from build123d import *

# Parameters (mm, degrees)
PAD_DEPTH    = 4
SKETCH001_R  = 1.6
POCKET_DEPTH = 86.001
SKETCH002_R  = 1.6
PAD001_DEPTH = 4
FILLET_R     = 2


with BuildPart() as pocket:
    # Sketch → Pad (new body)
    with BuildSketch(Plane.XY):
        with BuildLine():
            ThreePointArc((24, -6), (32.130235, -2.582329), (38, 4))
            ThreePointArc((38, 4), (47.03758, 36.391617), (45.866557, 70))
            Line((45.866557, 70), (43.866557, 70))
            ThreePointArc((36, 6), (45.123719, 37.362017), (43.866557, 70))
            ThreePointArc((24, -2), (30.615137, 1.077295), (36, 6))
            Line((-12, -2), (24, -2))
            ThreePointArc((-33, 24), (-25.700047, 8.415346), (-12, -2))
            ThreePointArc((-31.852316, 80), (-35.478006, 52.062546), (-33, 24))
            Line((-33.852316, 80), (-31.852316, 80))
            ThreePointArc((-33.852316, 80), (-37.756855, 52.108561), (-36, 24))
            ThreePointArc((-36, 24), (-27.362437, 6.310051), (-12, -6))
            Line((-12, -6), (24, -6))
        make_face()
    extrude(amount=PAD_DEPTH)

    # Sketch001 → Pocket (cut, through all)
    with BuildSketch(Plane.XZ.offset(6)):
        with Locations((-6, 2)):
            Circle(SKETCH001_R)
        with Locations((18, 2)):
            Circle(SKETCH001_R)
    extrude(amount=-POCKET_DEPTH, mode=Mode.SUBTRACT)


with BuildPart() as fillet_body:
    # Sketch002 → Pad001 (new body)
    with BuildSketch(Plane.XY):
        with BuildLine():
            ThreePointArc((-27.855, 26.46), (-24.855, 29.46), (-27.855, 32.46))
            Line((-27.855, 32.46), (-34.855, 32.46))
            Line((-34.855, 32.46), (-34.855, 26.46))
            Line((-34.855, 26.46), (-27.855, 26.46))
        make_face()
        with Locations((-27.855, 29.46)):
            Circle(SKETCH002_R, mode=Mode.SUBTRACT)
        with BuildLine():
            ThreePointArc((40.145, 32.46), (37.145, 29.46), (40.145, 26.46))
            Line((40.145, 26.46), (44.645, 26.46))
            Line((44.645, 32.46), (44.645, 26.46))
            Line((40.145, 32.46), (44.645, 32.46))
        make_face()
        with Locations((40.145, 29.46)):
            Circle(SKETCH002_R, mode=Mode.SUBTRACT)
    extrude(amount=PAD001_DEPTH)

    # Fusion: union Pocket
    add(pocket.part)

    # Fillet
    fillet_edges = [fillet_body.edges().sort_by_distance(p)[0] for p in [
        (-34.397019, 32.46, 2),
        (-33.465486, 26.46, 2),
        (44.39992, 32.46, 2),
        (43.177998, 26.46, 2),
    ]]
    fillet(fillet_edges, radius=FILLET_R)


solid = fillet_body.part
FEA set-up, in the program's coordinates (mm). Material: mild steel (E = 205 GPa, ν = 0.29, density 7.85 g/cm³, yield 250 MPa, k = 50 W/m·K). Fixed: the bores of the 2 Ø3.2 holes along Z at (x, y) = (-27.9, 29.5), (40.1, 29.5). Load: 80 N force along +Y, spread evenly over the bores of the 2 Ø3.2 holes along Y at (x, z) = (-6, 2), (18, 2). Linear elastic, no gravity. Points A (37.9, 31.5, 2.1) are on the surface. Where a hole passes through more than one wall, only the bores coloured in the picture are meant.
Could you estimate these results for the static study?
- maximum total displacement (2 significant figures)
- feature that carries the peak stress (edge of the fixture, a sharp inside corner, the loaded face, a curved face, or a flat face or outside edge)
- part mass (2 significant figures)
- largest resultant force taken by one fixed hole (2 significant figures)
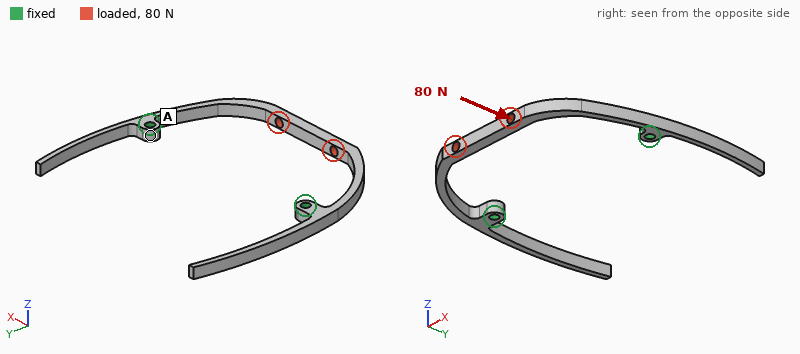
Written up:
29 µm
the loaded face
20 g
54 N
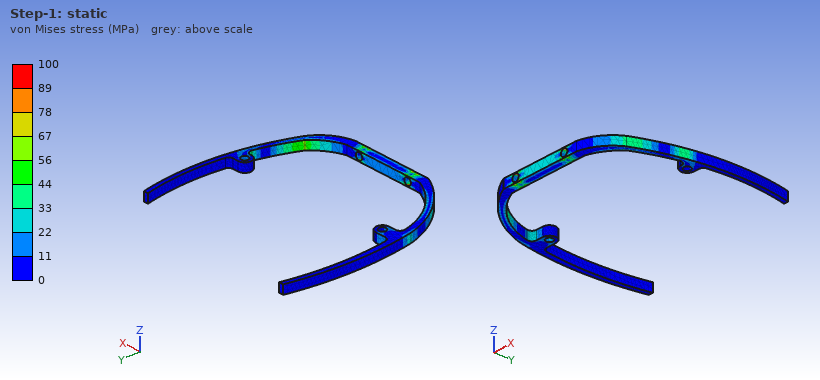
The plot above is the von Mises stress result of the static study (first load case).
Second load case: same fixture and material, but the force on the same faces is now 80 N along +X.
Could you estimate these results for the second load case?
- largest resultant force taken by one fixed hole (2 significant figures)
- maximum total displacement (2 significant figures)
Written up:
47 N
59 µm
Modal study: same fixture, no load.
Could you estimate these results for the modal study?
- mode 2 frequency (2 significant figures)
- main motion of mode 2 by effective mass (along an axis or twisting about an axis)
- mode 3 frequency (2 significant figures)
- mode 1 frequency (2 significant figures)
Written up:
1100 Hz
along Z
1100 Hz
950 Hz
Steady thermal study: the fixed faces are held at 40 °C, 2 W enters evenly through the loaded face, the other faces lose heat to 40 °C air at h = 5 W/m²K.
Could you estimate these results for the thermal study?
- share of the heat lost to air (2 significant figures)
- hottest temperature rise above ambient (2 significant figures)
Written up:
20 %
74 K
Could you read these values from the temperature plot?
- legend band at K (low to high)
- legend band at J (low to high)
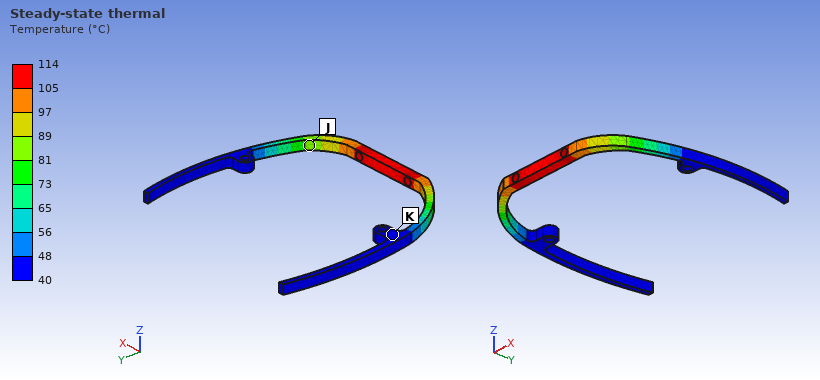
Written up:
40 to 48 °C
81 to 89 °C
